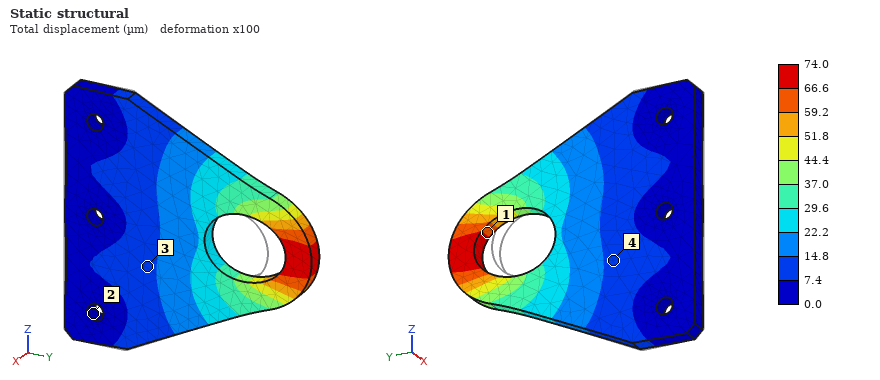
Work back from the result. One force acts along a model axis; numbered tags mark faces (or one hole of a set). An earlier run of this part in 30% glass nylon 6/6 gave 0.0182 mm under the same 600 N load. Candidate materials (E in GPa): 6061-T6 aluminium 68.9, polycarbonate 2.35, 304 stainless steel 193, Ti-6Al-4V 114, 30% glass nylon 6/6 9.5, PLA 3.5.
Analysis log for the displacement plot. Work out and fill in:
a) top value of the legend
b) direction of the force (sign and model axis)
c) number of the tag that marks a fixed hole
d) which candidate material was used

74.0 µm
+Y
2
polycarbonate
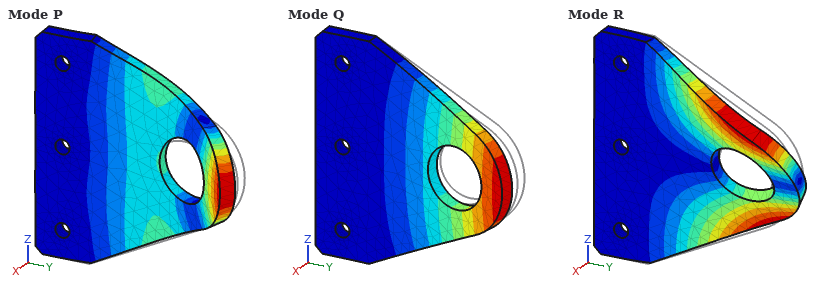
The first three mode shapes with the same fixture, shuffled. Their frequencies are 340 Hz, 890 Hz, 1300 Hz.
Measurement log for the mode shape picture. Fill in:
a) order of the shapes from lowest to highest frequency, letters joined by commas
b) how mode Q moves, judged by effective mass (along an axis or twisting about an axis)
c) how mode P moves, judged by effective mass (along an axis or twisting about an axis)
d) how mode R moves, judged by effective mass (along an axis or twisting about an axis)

Q, R, P
along X
along X
twisting about Y
